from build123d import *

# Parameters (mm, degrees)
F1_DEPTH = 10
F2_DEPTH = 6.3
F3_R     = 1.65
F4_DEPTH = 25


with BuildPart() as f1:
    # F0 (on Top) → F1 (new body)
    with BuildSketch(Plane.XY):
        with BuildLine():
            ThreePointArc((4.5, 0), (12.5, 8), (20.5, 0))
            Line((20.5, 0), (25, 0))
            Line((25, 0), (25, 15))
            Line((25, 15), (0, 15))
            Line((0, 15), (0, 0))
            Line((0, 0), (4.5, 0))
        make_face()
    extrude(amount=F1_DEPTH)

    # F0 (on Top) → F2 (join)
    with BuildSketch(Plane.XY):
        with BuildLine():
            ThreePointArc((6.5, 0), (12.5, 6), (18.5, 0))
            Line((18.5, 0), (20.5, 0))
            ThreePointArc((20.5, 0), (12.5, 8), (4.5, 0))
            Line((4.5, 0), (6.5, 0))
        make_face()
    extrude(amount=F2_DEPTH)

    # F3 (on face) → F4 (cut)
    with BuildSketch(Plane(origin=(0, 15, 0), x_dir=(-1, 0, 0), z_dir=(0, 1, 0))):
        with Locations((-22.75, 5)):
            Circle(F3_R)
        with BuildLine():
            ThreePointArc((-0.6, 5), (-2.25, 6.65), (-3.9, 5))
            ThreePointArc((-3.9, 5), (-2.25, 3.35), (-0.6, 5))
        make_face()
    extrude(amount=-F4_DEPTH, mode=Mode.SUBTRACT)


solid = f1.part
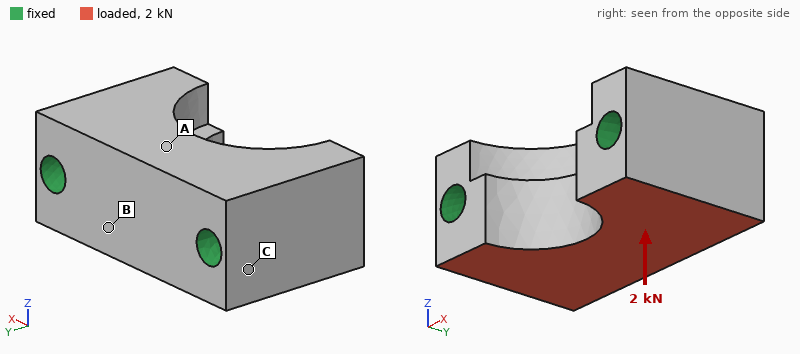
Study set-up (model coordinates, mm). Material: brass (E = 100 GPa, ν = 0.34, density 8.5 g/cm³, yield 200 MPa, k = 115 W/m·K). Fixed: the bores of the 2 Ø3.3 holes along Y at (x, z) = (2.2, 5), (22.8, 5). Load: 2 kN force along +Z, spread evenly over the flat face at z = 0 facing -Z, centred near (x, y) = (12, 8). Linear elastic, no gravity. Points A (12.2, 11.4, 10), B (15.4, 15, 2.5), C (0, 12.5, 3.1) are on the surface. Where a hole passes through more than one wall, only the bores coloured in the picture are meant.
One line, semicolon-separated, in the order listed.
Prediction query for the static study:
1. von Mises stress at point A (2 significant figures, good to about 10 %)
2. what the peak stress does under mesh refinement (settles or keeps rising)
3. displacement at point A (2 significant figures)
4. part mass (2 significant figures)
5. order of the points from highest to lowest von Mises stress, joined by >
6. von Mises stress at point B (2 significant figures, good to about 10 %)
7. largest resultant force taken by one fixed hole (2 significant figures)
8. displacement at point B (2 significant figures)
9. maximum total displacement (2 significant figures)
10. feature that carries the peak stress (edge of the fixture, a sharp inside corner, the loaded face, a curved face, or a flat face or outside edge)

11 MPa; keeps rising; 1.3 µm; 24 g; A > B > C; 6.8 MPa; 1.0 kN; 1.5 µm; 1.8 µm; edge of the fixture
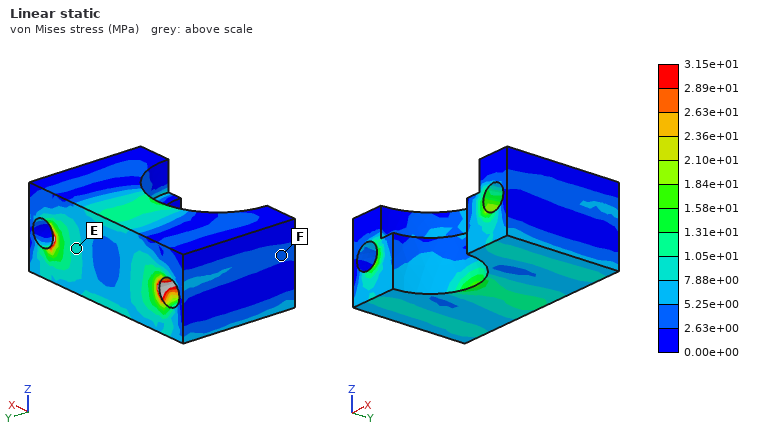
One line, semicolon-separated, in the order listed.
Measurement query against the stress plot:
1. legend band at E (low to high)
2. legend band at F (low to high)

7.88e+00 to 1.05e+01 MPa; 2.63e+00 to 5.25e+00 MPa
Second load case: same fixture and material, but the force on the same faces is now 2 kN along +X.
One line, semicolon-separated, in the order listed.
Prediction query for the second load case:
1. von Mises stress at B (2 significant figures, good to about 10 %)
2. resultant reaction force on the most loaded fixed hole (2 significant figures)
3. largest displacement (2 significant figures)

9.2 MPa; 1.1 kN; 1.8 µm
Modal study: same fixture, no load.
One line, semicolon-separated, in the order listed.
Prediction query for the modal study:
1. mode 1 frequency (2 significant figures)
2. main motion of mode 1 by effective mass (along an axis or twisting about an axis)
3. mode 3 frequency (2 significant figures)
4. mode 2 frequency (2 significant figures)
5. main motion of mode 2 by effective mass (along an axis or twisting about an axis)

40 kHz; along Z; 60 kHz; 51 kHz; along Y
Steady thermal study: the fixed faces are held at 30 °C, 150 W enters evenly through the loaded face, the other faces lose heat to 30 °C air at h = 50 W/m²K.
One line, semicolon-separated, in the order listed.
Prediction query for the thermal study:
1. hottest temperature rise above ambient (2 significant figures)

34 K
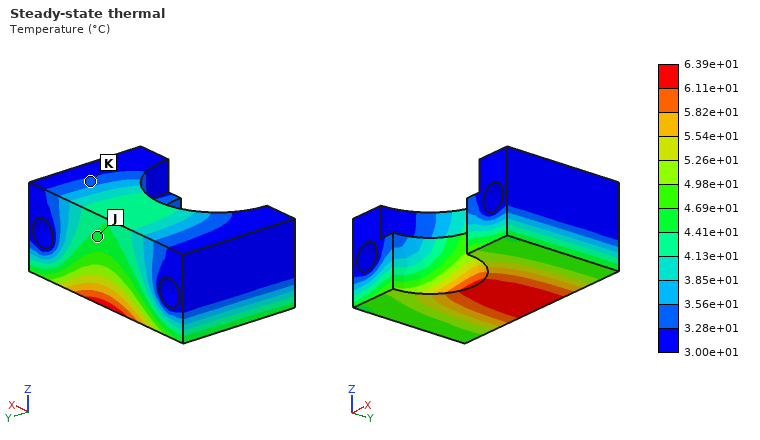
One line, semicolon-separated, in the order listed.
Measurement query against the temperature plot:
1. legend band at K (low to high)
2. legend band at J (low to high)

3.28e+01 to 3.56e+01 °C; 4.41e+01 to 4.69e+01 °C
